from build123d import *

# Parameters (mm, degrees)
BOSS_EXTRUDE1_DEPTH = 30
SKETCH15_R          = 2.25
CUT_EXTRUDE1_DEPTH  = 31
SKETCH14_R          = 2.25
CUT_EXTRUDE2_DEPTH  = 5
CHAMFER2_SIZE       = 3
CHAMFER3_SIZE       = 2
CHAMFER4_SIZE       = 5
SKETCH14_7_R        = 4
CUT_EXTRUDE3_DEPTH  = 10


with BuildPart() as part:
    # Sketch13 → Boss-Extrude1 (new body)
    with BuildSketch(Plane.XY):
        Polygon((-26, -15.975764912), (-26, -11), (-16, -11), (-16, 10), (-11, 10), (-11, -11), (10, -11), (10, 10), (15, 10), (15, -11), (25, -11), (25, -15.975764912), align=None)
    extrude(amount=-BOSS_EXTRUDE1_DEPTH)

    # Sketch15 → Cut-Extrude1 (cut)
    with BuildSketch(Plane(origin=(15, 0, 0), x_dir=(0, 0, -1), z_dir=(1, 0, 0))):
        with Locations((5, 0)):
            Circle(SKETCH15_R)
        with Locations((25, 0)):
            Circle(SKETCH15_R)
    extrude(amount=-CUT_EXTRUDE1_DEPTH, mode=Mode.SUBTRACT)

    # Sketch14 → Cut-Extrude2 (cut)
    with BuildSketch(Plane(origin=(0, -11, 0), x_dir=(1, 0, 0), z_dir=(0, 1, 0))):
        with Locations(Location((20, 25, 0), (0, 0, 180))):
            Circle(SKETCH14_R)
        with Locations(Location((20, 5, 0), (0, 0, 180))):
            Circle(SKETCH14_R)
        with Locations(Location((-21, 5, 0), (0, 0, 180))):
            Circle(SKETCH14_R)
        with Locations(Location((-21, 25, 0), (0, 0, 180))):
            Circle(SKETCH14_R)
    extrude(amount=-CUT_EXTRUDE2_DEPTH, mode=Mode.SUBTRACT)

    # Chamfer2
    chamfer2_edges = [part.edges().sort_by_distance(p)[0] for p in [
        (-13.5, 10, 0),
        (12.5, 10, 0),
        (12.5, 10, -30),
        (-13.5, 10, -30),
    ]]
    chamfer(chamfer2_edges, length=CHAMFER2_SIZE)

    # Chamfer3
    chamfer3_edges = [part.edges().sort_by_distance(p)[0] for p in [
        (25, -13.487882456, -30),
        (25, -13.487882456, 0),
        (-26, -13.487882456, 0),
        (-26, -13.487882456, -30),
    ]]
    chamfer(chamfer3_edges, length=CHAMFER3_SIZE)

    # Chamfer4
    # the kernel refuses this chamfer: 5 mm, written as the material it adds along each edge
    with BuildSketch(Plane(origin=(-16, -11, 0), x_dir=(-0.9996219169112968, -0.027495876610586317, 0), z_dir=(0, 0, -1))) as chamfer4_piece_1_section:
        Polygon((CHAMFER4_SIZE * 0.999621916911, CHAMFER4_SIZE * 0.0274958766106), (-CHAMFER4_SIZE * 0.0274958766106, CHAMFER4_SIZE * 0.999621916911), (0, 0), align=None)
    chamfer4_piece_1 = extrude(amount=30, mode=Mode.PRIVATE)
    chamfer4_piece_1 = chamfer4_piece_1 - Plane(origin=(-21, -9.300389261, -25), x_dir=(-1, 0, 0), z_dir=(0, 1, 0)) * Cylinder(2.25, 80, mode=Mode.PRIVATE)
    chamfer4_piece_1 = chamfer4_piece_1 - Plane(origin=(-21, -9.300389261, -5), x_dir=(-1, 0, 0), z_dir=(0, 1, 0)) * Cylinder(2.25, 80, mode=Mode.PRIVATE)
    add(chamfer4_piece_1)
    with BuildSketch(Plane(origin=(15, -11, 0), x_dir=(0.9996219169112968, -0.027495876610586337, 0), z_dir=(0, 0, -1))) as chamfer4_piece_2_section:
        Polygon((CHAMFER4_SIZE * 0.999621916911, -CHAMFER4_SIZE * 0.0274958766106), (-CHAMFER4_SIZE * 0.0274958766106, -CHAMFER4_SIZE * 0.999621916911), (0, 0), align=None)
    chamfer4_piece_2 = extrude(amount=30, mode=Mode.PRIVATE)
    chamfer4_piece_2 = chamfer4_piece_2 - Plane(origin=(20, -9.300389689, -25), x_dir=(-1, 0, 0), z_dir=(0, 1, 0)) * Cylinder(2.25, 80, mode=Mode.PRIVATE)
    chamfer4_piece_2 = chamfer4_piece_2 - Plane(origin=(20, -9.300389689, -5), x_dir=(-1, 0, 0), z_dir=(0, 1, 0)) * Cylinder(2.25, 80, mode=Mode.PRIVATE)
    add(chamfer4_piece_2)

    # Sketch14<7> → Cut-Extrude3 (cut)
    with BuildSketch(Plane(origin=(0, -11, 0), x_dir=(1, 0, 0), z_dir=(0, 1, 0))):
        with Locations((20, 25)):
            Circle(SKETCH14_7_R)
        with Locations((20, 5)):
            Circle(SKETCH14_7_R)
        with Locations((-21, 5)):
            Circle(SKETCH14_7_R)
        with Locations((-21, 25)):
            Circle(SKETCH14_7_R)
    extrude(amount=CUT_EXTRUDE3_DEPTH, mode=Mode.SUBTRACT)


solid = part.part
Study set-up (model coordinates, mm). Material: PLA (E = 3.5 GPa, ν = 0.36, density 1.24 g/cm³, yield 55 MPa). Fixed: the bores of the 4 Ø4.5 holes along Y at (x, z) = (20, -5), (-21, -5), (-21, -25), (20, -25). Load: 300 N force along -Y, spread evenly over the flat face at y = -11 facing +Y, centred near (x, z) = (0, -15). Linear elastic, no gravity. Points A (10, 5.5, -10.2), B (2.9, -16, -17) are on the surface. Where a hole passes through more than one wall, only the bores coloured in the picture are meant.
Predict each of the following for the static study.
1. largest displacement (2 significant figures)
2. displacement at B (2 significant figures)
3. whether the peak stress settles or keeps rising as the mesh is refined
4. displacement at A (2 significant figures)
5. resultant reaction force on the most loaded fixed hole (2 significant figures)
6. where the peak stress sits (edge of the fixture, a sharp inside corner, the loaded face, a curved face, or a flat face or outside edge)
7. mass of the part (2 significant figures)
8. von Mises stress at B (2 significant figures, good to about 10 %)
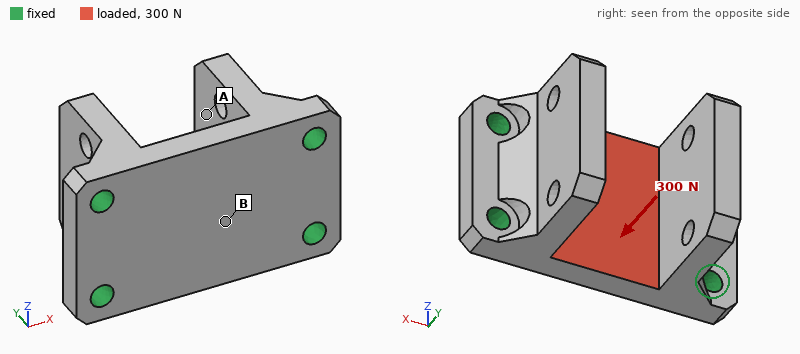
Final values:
0.11 mm
0.067 mm
keeps rising
0.090 mm
75 N
edge of the fixture
17 g
4.8 MPa
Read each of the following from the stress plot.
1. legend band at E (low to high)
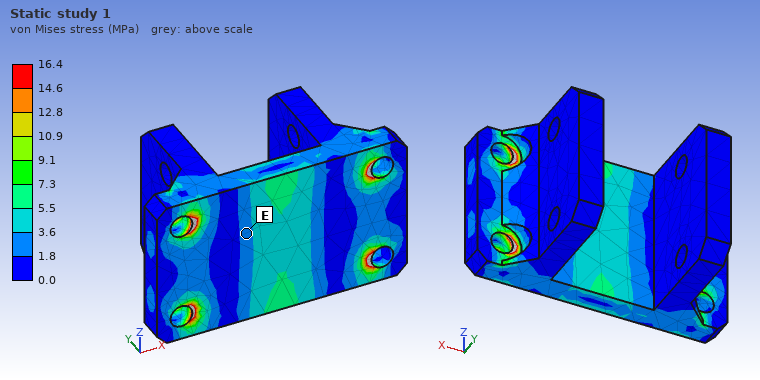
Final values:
1.8 to 3.6 MPa
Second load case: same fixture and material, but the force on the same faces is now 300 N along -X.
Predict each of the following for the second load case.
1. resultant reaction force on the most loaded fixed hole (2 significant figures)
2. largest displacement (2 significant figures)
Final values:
77 N
6.2 µm
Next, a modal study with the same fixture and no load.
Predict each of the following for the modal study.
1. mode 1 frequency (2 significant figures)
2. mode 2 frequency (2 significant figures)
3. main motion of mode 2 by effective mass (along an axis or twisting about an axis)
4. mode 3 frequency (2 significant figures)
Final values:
2400 Hz
3000 Hz
along X
4500 Hz
